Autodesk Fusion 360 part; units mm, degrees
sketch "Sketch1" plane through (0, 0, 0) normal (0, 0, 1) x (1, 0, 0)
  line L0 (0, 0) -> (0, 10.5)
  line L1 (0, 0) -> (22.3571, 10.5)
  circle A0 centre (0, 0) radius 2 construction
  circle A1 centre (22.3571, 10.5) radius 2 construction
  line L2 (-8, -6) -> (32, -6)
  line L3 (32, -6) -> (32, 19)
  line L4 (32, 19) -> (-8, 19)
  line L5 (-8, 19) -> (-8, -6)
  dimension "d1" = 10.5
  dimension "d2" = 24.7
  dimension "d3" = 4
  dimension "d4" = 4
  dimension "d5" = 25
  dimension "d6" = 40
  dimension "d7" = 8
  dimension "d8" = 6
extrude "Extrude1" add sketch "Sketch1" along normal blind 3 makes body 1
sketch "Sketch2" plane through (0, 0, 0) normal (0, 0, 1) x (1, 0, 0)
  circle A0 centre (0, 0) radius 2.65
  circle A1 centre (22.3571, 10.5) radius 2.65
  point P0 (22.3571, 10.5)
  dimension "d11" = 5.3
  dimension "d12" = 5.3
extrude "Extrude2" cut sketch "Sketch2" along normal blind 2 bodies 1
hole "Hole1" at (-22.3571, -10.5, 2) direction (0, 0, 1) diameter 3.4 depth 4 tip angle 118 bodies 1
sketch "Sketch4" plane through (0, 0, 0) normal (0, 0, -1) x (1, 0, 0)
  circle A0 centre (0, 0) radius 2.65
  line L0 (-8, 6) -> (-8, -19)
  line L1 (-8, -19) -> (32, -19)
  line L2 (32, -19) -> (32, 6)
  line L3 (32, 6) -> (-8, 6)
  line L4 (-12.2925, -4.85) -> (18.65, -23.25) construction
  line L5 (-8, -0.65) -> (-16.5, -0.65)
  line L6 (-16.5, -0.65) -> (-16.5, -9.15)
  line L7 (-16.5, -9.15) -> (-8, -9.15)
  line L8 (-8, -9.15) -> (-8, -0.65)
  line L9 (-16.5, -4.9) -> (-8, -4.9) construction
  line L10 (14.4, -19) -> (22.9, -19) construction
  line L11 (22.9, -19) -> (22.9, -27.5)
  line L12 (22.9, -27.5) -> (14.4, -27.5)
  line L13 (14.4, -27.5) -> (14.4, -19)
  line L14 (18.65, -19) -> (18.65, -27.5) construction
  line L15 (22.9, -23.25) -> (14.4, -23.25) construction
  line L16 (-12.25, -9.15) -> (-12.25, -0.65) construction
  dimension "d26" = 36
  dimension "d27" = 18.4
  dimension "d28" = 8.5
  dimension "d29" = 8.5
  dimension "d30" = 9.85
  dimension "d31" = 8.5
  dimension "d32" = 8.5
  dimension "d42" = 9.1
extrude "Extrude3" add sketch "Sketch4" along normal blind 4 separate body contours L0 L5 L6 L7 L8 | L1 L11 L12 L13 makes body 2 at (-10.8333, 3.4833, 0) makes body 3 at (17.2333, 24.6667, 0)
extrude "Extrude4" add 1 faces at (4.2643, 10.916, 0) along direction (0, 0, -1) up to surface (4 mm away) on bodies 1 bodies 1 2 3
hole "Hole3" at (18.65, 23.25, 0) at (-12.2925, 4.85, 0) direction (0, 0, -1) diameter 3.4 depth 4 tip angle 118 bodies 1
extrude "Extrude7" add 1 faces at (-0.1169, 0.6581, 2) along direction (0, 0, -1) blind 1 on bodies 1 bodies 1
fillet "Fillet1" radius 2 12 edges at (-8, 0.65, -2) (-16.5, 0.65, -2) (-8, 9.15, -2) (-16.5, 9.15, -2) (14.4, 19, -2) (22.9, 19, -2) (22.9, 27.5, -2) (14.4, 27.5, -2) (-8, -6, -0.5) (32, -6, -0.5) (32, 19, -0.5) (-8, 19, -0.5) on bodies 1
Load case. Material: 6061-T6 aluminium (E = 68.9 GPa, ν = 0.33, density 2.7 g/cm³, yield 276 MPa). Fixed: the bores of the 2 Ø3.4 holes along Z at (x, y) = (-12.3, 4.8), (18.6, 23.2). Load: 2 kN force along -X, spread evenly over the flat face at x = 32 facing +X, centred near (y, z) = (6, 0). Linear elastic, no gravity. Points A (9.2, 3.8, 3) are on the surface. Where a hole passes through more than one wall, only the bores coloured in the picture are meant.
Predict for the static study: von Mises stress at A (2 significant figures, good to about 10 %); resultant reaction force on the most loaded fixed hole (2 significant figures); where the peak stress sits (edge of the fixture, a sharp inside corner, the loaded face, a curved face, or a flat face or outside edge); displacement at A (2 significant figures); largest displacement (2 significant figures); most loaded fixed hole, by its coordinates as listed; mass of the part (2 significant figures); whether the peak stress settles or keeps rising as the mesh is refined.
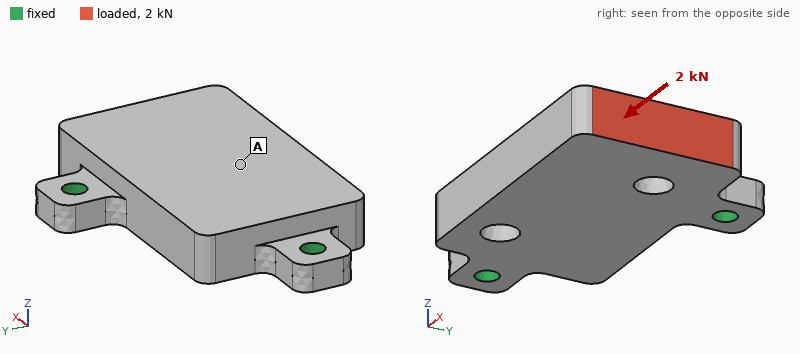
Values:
12 MPa
1.4 kN
edge of the fixture
15 µm
29 µm
(-12.3, 4.8)
20 g
keeps rising
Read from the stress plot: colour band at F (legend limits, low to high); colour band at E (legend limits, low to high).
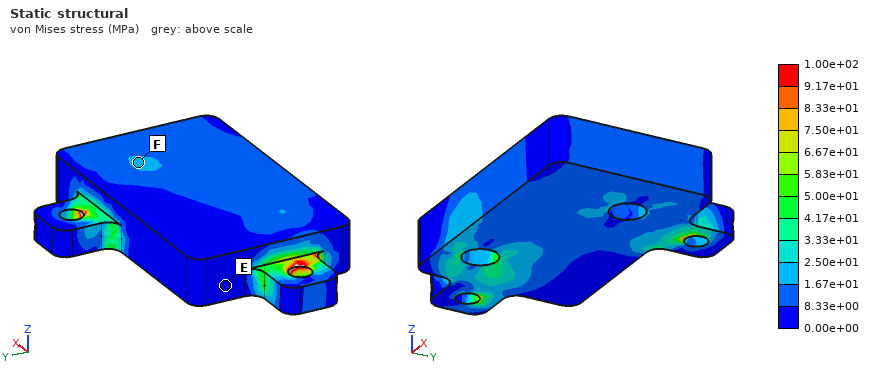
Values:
1.67e+01 to 2.50e+01 MPa
0.00e+00 to 8.33e+00 MPa
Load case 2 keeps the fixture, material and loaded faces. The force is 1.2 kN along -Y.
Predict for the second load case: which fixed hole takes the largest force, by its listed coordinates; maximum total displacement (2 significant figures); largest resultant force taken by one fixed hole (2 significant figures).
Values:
(18.6, 23.2)
40 µm
1.5 kN
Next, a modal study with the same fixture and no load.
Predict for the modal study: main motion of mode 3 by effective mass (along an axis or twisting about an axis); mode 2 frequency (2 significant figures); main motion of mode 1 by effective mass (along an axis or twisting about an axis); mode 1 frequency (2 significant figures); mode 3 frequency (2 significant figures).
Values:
along Z
13 kHz
along Z
3400 Hz
16 kHz
